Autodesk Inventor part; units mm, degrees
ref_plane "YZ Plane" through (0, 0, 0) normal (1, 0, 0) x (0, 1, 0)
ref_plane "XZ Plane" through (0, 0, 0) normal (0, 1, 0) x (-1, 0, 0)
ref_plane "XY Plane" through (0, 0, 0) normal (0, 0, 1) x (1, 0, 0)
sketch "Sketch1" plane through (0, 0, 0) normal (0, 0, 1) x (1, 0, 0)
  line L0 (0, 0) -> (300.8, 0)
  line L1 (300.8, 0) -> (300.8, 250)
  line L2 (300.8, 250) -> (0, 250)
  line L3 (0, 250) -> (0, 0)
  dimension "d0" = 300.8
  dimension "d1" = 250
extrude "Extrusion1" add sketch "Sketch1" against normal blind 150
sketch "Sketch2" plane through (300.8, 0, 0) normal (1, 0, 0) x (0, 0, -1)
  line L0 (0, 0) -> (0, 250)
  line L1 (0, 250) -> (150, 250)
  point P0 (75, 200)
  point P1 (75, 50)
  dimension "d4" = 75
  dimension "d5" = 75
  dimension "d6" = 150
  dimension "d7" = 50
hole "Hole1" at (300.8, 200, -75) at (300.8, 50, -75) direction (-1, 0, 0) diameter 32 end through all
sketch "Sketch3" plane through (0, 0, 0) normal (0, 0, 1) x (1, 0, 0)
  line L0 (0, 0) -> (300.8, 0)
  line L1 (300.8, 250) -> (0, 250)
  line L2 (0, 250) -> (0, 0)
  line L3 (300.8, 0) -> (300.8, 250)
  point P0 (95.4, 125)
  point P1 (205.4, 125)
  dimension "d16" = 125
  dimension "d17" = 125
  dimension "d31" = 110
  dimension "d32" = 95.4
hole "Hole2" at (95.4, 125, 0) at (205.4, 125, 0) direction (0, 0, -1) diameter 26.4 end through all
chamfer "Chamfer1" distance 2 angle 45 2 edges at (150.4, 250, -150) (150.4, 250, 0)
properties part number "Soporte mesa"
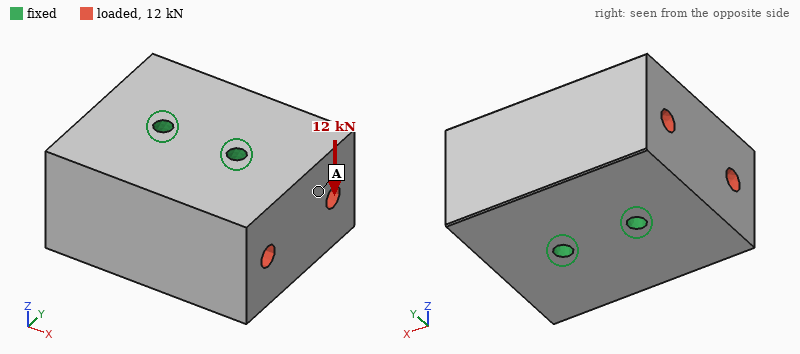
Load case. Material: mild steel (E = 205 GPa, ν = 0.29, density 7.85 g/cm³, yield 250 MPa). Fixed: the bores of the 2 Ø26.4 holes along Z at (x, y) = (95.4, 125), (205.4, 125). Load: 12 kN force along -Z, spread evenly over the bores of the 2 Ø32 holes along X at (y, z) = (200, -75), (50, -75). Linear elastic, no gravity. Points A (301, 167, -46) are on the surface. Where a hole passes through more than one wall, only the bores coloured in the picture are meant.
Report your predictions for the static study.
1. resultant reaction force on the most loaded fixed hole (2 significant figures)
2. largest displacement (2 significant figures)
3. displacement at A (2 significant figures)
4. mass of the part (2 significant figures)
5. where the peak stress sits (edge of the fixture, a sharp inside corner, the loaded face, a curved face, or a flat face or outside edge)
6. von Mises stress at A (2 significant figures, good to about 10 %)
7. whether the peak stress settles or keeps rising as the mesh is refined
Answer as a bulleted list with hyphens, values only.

- 6.0 kN
- 0.36 µm
- 0.22 µm
- 83 kg
- edge of the fixture
- 0.17 MPa
- keeps rising
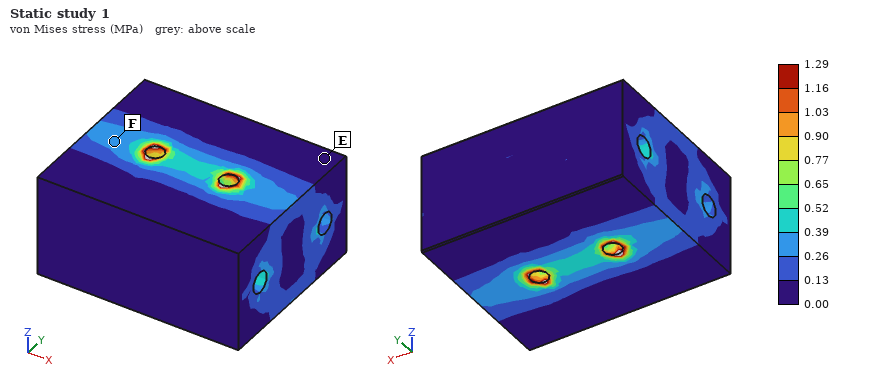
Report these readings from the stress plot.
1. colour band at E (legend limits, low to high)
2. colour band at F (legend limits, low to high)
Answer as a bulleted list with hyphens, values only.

- 0.00 to 0.13 MPa
- 0.26 to 0.39 MPa
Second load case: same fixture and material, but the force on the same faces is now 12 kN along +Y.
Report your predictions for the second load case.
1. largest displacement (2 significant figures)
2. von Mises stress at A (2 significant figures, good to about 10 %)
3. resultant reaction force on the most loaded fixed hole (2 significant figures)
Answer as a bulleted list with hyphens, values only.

- 0.22 µm
- 0.13 MPa
- 6.0 kN
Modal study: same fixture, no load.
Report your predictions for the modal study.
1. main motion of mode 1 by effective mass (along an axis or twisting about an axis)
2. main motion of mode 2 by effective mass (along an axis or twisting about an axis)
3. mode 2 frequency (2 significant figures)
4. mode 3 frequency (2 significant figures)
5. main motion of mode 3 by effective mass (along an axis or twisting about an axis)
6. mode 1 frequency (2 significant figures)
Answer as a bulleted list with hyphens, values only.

- twisting about Z
- twisting about X
- 3400 Hz
- 3900 Hz
- twisting about Y
- 2900 Hz
